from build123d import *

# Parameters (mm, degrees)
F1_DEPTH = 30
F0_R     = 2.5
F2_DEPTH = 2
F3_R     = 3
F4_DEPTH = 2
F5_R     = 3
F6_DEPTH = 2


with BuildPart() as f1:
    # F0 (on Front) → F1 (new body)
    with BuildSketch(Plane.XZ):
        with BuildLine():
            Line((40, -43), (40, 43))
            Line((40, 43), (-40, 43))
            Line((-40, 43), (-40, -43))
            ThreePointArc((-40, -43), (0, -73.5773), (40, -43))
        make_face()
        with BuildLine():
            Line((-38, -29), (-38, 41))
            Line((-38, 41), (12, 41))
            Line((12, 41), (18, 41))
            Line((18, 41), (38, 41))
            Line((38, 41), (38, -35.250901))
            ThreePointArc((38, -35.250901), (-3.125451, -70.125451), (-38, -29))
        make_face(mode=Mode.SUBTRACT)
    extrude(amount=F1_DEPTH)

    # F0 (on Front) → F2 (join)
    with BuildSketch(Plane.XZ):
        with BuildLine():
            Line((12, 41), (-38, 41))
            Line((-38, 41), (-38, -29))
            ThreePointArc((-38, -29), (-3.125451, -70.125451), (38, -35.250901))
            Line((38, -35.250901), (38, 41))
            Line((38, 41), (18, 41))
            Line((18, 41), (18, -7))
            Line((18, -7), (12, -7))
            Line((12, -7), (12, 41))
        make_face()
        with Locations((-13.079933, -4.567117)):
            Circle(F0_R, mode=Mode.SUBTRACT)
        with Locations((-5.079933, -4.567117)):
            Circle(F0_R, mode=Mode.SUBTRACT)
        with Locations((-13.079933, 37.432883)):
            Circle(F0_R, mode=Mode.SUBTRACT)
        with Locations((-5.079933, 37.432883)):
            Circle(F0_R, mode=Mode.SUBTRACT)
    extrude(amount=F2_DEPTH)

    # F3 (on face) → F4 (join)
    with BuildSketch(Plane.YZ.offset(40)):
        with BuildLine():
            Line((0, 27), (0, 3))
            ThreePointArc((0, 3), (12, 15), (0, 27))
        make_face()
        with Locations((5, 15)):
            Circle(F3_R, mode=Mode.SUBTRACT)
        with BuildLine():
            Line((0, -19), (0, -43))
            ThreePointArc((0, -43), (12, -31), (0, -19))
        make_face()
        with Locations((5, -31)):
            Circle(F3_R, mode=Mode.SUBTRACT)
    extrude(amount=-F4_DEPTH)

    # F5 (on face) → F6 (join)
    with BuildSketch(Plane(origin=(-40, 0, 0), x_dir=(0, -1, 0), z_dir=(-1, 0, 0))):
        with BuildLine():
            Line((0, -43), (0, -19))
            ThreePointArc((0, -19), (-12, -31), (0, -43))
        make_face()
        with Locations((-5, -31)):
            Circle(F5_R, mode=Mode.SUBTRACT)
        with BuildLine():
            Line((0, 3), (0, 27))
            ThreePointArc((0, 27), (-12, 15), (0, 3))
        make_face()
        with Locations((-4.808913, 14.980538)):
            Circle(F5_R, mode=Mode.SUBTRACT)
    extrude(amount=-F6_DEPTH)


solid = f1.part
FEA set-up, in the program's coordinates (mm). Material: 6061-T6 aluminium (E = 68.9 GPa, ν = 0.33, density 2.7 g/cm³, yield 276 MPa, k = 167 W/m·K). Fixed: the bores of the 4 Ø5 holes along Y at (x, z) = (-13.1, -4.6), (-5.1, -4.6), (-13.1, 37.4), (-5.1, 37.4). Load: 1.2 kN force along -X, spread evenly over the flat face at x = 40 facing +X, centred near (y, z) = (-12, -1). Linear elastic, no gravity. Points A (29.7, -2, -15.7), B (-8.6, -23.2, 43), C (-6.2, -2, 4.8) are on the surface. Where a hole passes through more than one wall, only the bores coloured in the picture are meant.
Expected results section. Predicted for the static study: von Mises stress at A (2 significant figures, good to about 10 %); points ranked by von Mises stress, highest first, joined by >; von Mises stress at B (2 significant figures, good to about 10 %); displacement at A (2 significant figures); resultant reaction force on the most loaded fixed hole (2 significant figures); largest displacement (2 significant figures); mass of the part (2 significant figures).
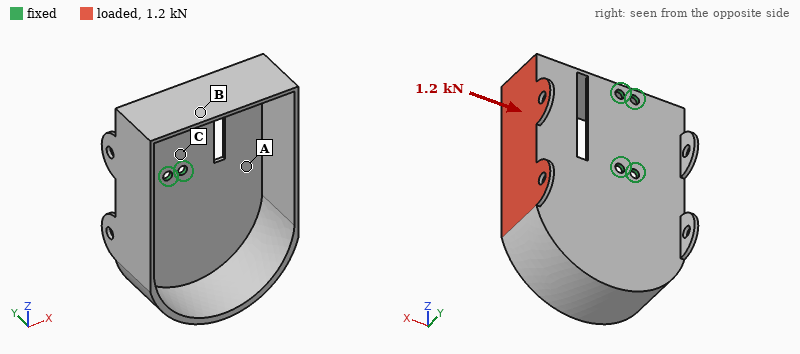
68 MPa
A > B > C
45 MPa
0.51 mm
860 N
1.5 mm
110 g
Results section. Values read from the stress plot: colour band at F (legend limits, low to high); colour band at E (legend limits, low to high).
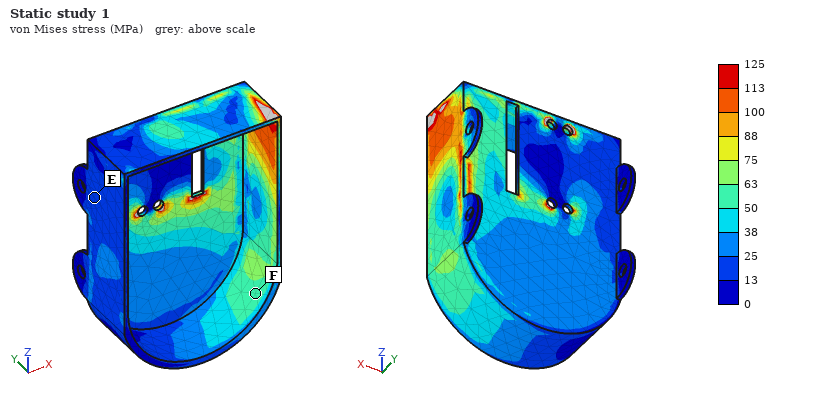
50 to 63 MPa
13 to 25 MPa
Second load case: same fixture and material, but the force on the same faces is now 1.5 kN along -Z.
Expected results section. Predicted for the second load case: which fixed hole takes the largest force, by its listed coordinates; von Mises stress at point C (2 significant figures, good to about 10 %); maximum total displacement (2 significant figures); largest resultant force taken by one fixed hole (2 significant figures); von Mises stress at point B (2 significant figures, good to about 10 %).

(-5.1, -4.6)
26 MPa
1.6 mm
1.8 kN
21 MPa
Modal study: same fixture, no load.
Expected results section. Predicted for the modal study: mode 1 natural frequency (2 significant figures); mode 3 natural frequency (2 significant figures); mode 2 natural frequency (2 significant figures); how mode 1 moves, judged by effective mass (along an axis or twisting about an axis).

340 Hz
1500 Hz
540 Hz
along Y
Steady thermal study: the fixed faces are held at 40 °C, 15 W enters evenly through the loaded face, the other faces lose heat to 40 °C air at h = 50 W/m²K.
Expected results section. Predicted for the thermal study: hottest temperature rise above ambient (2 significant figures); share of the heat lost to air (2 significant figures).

18 K
64 %
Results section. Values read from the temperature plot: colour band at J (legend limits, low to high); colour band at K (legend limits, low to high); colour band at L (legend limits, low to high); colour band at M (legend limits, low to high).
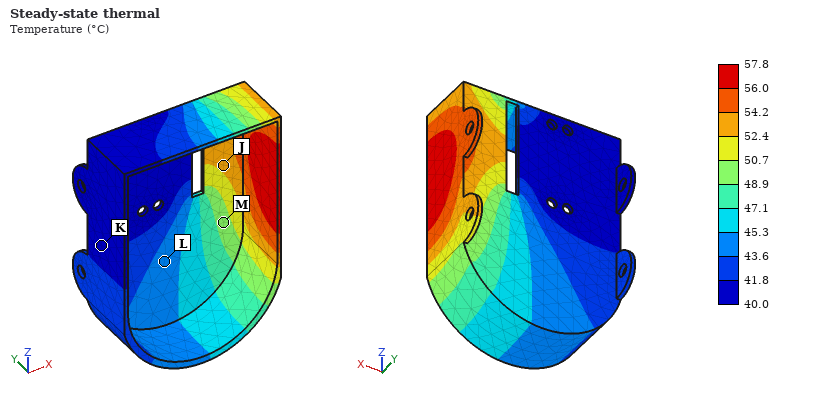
52.4 to 54.2 °C
40.0 to 41.8 °C
43.6 to 45.3 °C
48.9 to 50.7 °C
